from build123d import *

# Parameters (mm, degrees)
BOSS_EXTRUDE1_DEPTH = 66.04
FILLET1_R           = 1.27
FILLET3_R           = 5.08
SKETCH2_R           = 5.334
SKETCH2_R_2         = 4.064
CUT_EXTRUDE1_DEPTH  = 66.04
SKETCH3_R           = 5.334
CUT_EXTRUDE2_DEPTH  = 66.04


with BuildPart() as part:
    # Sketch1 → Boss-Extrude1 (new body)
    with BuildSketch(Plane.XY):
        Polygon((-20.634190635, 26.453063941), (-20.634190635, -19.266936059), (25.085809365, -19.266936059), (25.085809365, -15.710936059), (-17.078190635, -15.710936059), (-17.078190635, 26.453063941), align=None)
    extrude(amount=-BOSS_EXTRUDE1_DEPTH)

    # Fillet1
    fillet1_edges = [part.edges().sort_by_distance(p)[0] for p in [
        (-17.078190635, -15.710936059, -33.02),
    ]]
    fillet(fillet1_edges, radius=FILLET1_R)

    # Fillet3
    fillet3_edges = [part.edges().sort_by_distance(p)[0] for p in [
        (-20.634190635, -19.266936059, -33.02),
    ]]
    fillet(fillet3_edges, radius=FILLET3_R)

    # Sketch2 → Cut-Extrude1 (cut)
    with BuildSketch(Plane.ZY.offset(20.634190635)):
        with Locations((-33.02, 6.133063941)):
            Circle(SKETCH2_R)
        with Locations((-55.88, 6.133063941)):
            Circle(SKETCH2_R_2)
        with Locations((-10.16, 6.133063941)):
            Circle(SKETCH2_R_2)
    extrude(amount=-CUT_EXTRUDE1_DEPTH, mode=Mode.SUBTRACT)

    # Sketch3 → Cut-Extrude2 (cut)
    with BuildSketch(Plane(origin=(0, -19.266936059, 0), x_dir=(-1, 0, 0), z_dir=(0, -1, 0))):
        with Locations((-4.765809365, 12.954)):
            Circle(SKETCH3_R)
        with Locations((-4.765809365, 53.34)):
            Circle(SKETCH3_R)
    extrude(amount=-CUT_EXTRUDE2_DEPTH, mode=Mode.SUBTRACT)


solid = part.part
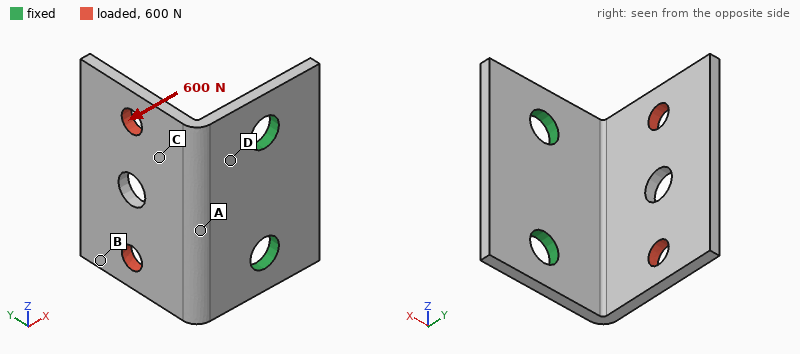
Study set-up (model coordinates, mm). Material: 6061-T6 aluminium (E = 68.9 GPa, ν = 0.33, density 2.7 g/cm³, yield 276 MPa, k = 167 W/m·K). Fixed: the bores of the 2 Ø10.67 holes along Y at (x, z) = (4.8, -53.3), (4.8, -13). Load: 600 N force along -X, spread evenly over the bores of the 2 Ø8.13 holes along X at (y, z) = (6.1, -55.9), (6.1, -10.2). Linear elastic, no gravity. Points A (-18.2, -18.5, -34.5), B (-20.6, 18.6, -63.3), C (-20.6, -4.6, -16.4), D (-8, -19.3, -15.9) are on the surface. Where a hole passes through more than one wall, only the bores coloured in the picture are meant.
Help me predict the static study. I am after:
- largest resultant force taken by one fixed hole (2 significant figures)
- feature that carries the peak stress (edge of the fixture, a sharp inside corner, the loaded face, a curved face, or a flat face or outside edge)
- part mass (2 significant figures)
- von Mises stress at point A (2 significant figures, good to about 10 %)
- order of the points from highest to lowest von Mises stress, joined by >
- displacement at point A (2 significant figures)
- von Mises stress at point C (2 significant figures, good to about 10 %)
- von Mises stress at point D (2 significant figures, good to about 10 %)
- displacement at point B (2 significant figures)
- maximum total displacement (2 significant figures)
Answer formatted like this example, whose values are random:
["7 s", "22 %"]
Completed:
["300 N", "a flat face or outside edge", "51 g", "65 MPa", "D > A > C > B", "0.15 mm", "43 MPa", "91 MPa", "0.84 mm", "1.0 mm"]
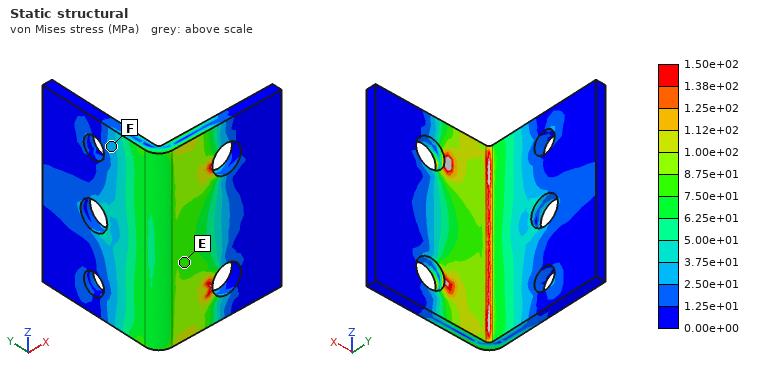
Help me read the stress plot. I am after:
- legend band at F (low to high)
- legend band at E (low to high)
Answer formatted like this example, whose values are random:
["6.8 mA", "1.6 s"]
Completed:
["2.50e+01 to 3.75e+01 MPa", "7.50e+01 to 8.75e+01 MPa"]
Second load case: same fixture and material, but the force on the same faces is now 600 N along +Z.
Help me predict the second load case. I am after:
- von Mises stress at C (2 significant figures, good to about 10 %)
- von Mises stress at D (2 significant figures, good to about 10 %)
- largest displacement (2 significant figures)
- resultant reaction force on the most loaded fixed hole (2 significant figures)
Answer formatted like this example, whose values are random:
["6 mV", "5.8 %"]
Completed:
["10 MPa", "30 MPa", "0.18 mm", "510 N"]
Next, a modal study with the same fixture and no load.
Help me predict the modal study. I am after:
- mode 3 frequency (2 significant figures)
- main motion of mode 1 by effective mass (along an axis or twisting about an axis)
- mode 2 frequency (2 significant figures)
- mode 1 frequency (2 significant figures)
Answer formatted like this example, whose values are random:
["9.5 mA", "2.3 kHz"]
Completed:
["2900 Hz", "along X", "1800 Hz", "910 Hz"]
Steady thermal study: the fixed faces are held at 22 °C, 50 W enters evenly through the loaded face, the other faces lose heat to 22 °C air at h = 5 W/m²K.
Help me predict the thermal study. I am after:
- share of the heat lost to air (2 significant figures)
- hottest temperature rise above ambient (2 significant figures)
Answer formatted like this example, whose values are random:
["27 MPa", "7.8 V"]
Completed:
["3.4 %", "66 K"]
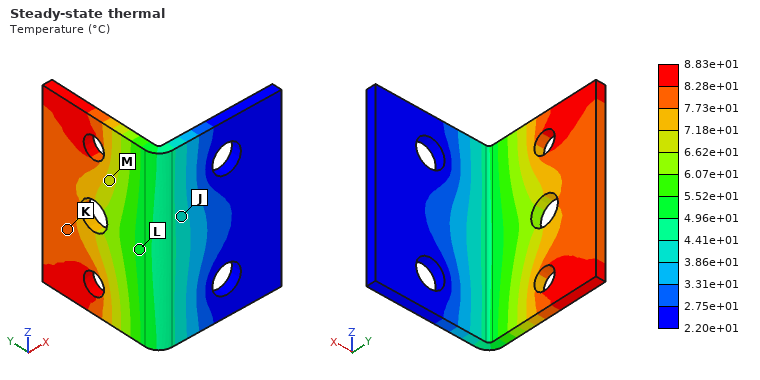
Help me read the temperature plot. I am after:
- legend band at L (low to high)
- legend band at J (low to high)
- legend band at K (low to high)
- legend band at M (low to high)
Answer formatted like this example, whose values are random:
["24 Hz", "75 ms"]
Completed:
["4.96e+01 to 5.52e+01 °C", "3.86e+01 to 4.41e+01 °C", "7.73e+01 to 8.28e+01 °C", "6.62e+01 to 7.18e+01 °C"]
